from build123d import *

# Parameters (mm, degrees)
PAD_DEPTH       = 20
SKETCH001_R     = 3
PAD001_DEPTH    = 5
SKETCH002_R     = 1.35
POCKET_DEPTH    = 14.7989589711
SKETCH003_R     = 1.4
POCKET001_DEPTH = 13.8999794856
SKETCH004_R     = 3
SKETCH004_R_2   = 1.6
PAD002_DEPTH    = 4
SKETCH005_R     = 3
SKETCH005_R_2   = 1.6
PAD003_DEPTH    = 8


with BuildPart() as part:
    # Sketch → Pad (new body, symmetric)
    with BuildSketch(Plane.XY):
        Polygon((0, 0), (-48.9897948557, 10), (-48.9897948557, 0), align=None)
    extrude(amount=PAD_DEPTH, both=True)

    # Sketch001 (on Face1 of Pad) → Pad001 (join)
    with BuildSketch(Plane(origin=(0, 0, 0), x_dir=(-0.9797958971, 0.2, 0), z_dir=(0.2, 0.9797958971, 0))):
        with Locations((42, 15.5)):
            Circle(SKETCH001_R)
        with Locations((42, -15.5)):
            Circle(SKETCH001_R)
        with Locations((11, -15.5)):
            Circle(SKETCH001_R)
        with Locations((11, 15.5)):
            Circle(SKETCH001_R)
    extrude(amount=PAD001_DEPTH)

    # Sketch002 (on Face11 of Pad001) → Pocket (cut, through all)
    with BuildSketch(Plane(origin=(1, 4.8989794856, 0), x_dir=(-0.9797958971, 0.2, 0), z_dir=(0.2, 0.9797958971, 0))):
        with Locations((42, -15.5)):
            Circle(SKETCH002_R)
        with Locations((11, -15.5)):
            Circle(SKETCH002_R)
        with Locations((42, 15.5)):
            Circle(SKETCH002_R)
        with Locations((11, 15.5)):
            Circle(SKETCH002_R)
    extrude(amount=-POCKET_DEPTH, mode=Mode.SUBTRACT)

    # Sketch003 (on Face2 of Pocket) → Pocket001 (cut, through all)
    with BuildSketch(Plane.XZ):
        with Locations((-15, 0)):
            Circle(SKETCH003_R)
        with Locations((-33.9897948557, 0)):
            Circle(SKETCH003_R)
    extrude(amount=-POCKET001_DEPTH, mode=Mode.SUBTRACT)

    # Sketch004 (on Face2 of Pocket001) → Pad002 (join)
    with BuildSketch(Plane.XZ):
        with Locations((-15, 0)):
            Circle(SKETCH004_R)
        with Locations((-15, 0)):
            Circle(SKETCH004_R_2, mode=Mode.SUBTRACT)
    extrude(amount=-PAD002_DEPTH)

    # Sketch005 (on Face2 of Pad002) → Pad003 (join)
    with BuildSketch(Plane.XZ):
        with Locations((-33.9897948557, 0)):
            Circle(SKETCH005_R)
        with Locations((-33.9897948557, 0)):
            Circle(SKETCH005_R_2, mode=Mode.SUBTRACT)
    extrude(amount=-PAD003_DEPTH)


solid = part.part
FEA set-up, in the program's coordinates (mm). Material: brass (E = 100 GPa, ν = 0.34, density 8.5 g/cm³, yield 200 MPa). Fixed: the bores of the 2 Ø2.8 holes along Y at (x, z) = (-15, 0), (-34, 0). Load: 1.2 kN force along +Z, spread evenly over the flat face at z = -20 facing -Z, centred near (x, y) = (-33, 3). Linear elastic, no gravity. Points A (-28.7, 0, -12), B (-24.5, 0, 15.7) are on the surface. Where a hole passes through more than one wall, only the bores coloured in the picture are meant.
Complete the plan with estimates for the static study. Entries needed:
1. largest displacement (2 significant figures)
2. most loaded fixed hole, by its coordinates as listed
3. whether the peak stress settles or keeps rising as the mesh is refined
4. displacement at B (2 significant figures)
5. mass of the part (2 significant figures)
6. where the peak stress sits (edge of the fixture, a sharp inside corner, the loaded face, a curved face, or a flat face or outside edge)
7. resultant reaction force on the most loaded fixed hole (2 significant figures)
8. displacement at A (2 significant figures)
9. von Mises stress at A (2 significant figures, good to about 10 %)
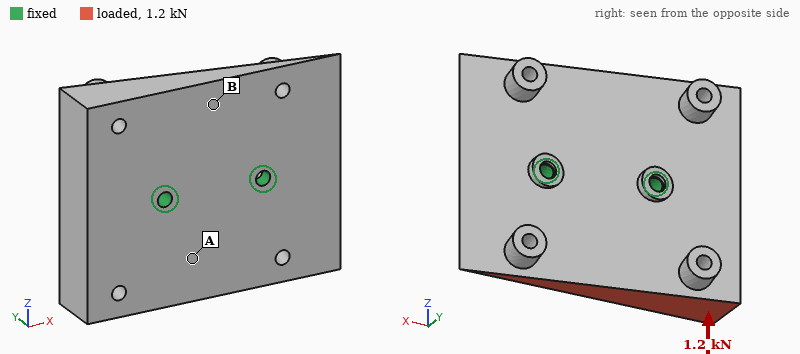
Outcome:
3.3 µm
(-34, 0)
keeps rising
0.80 µm
86 g
edge of the fixture
1.1 kN
1.1 µm
6.0 MPa
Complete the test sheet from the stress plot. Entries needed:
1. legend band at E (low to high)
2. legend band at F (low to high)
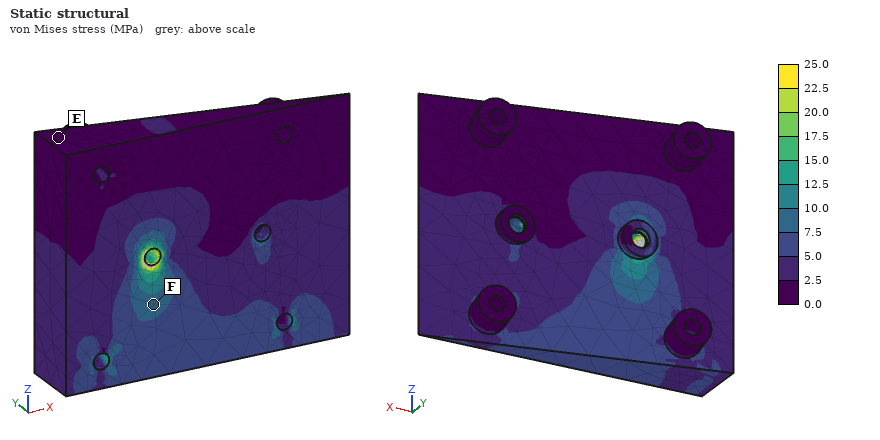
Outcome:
0.0 to 2.5 MPa
7.5 to 10.0 MPa
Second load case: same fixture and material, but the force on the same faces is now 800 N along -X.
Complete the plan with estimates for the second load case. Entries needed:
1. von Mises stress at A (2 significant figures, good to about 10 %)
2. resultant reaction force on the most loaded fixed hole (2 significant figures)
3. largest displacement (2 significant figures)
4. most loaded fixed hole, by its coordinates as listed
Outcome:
12 MPa
940 N
12 µm
(-34, 0)
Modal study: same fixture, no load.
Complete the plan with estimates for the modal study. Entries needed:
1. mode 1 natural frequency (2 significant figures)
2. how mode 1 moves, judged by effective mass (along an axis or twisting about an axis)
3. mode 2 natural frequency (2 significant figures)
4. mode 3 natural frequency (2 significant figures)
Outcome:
4900 Hz
twisting about X
6000 Hz
6400 Hz
